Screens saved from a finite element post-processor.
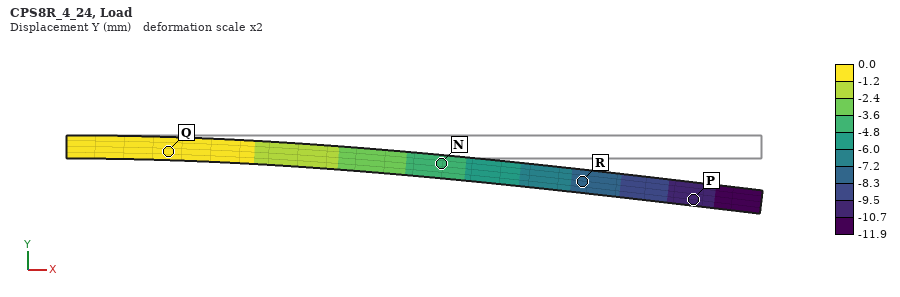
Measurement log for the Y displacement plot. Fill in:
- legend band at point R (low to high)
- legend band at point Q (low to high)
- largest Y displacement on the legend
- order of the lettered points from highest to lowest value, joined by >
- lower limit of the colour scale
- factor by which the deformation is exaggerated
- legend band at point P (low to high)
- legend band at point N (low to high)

-8.3 to -7.2 mm
-1.2 to 0.0 mm
0.0 mm
Q > N > R > P
-11.9 mm
2
-10.7 to -9.5 mm
-4.8 to -3.6 mm
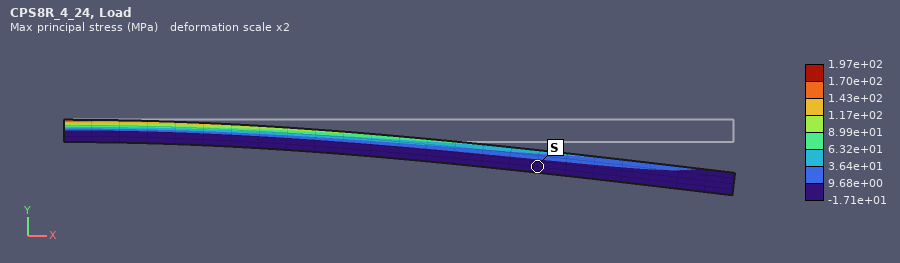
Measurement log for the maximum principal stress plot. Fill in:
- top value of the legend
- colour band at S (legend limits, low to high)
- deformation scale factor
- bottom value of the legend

1.97e+02 MPa
-1.71e+01 to 9.68e+00 MPa
2
-1.71e+01 MPa
